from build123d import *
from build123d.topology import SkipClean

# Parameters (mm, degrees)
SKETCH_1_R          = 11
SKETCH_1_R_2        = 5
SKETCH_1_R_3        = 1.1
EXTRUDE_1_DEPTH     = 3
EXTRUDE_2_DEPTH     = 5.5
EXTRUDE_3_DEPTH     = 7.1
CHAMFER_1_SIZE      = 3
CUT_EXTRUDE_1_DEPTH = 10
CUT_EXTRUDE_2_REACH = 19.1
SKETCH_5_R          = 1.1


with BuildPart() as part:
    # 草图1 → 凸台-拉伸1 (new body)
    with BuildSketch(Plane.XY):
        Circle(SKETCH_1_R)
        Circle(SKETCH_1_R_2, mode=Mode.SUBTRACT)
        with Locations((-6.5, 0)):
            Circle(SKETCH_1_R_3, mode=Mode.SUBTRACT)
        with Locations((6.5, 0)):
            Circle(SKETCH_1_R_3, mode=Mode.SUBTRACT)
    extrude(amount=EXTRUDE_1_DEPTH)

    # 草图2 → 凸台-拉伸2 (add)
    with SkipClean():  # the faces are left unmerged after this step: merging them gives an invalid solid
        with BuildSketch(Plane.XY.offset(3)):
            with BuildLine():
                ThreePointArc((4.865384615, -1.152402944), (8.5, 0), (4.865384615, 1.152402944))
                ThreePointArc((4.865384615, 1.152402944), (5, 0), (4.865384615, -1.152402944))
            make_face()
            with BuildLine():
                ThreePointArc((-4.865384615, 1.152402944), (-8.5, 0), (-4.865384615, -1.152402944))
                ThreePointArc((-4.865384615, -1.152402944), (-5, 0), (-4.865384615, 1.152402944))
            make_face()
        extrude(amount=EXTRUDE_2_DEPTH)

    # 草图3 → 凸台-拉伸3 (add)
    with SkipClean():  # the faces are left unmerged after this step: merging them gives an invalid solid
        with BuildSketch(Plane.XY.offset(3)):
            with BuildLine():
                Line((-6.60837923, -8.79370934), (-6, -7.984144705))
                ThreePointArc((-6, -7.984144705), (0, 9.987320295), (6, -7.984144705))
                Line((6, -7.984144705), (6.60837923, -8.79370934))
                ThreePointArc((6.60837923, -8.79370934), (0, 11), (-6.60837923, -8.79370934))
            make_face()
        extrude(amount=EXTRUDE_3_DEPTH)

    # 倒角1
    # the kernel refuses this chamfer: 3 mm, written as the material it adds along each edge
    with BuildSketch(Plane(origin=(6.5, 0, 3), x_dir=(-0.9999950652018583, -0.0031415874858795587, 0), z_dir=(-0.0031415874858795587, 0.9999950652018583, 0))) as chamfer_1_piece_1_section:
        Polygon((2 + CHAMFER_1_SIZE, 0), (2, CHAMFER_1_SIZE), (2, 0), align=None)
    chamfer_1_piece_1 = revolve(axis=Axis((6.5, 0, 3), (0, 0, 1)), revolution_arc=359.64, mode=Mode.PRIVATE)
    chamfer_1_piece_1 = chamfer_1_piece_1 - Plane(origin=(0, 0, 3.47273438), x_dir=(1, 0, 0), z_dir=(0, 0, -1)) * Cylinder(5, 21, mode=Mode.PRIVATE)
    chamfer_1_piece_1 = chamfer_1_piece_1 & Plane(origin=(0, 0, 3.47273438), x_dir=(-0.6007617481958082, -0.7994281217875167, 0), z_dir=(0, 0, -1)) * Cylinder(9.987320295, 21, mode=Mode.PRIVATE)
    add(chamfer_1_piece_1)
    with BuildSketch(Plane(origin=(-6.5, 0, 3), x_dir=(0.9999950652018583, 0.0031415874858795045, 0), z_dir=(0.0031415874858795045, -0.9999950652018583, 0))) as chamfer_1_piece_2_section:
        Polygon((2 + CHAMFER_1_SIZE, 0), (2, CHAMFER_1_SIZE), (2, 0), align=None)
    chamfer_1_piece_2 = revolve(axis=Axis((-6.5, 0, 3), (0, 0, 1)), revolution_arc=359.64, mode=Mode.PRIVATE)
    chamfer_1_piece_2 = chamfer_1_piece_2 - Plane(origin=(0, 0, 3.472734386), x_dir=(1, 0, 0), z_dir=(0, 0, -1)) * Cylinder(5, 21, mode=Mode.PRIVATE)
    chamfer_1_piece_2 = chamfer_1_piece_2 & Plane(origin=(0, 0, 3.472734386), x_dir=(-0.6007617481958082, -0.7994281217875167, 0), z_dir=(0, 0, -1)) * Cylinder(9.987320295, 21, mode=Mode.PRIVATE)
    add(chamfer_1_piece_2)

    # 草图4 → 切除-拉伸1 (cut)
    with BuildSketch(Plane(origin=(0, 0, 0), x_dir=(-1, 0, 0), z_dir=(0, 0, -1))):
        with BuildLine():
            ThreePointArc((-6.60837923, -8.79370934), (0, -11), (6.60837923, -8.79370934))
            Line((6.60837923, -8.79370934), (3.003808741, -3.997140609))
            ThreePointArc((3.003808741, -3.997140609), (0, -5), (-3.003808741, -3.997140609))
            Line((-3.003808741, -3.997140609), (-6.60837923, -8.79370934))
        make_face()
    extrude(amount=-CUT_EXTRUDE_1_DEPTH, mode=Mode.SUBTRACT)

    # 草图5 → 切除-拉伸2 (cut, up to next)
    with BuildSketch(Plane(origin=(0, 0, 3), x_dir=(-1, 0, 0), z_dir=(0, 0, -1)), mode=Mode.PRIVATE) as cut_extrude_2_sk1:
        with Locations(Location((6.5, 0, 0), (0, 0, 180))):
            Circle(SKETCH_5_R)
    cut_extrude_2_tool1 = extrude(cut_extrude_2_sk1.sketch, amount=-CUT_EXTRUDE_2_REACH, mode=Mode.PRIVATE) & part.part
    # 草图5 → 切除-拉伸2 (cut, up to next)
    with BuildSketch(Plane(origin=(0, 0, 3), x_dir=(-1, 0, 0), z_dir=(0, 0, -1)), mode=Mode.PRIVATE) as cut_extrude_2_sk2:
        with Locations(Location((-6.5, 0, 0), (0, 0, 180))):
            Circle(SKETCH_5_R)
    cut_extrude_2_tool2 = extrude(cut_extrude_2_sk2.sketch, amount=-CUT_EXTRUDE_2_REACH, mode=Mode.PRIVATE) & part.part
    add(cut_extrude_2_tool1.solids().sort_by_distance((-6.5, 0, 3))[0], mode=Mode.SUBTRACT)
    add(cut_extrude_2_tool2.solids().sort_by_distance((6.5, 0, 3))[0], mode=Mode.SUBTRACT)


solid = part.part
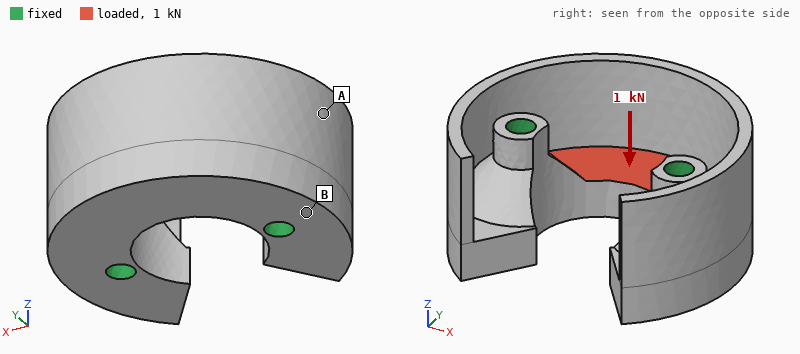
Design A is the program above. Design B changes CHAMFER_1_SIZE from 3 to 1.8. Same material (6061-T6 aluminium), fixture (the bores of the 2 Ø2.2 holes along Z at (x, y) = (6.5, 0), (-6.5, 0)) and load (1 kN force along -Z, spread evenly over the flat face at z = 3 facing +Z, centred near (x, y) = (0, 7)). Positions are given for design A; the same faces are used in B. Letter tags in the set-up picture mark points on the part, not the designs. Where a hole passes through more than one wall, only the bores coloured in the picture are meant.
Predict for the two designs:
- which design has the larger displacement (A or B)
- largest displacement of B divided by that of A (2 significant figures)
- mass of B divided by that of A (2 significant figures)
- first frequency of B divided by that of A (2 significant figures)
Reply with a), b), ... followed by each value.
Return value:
a) B
b) 1.2
c) 0.94
d) 0.83
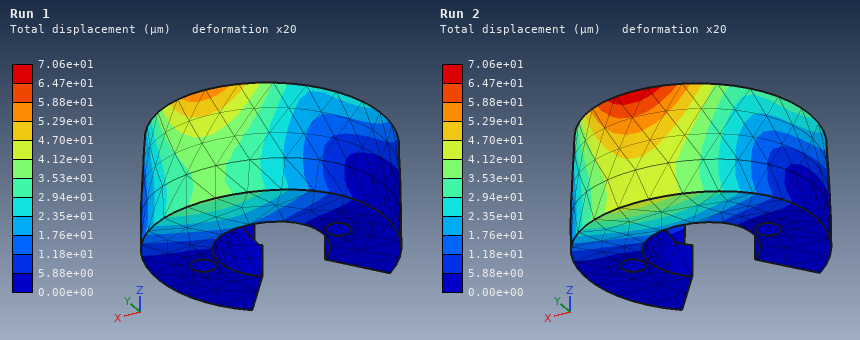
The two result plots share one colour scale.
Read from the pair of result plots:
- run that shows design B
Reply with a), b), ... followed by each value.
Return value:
a) Run 2
